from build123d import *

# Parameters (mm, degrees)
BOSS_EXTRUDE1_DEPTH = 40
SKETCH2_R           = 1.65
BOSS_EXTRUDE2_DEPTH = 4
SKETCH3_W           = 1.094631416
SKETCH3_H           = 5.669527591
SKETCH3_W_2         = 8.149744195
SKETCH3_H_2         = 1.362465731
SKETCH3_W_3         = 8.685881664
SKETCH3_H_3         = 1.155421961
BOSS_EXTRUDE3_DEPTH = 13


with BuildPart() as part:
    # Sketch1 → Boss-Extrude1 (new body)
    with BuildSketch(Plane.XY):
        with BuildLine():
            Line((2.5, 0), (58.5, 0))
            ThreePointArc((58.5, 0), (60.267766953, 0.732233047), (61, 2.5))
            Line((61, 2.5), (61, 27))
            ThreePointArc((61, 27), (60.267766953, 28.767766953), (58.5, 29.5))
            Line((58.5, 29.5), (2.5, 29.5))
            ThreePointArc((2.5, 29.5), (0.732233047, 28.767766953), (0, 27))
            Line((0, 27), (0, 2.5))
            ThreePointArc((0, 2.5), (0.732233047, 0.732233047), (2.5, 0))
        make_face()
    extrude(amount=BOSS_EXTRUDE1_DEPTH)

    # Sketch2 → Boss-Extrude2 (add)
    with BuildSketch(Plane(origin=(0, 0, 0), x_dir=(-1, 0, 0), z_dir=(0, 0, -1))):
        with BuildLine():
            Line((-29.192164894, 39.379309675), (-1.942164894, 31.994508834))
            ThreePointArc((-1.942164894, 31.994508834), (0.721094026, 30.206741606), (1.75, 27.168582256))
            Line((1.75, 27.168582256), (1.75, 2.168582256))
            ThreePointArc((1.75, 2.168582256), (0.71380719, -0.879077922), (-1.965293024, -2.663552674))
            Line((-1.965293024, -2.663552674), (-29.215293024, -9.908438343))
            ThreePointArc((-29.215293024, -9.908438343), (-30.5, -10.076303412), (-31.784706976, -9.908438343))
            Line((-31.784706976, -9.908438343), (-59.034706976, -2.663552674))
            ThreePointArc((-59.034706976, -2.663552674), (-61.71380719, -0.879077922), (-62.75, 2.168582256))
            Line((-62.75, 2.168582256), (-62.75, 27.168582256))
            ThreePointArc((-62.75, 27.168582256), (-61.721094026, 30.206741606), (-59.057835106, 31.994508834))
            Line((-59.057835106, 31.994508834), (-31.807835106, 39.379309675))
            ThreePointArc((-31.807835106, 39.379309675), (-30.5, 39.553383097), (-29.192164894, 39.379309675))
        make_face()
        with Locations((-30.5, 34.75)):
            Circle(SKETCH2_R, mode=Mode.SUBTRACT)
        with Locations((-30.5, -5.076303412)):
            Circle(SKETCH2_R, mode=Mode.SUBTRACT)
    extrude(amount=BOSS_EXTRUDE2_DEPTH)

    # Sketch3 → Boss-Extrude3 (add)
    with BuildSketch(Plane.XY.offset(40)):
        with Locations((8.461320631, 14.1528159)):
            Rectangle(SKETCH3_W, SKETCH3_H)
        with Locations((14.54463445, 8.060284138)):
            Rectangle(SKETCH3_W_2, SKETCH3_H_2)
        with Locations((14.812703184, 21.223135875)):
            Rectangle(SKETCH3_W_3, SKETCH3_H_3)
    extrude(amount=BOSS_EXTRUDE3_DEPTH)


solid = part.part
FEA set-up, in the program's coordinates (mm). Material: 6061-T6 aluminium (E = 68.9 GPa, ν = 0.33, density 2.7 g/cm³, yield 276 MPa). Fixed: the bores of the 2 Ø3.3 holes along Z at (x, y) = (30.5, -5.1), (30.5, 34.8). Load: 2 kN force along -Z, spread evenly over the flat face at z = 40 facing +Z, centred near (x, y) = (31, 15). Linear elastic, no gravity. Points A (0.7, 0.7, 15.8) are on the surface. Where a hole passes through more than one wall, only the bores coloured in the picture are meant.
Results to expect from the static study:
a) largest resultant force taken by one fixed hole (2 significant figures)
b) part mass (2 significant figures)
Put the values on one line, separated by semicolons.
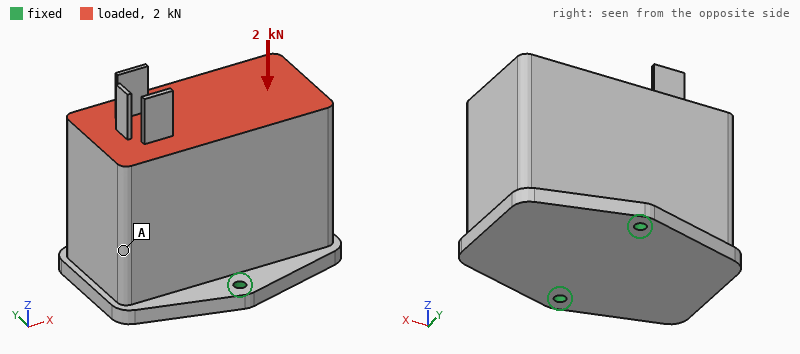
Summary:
1.1 kN; 220 g
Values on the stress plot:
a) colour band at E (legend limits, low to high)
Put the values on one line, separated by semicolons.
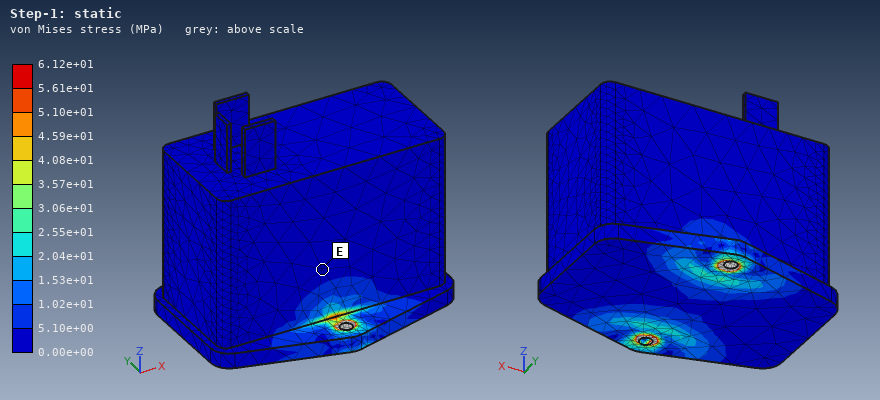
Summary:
0.00e+00 to 5.10e+00 MPa
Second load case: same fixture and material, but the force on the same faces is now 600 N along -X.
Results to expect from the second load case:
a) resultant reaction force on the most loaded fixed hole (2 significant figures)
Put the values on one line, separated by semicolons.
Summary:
300 N
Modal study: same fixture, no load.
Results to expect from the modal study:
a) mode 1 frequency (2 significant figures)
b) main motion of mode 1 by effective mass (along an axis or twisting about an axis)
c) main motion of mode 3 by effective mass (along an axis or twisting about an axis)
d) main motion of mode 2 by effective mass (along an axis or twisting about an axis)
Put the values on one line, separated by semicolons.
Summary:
710 Hz; along X; along Z; along Y
